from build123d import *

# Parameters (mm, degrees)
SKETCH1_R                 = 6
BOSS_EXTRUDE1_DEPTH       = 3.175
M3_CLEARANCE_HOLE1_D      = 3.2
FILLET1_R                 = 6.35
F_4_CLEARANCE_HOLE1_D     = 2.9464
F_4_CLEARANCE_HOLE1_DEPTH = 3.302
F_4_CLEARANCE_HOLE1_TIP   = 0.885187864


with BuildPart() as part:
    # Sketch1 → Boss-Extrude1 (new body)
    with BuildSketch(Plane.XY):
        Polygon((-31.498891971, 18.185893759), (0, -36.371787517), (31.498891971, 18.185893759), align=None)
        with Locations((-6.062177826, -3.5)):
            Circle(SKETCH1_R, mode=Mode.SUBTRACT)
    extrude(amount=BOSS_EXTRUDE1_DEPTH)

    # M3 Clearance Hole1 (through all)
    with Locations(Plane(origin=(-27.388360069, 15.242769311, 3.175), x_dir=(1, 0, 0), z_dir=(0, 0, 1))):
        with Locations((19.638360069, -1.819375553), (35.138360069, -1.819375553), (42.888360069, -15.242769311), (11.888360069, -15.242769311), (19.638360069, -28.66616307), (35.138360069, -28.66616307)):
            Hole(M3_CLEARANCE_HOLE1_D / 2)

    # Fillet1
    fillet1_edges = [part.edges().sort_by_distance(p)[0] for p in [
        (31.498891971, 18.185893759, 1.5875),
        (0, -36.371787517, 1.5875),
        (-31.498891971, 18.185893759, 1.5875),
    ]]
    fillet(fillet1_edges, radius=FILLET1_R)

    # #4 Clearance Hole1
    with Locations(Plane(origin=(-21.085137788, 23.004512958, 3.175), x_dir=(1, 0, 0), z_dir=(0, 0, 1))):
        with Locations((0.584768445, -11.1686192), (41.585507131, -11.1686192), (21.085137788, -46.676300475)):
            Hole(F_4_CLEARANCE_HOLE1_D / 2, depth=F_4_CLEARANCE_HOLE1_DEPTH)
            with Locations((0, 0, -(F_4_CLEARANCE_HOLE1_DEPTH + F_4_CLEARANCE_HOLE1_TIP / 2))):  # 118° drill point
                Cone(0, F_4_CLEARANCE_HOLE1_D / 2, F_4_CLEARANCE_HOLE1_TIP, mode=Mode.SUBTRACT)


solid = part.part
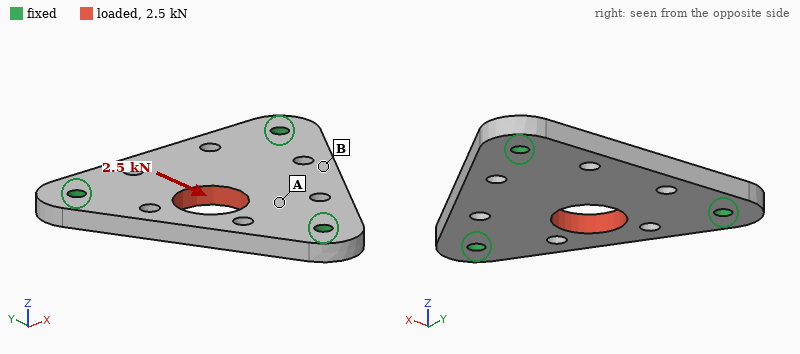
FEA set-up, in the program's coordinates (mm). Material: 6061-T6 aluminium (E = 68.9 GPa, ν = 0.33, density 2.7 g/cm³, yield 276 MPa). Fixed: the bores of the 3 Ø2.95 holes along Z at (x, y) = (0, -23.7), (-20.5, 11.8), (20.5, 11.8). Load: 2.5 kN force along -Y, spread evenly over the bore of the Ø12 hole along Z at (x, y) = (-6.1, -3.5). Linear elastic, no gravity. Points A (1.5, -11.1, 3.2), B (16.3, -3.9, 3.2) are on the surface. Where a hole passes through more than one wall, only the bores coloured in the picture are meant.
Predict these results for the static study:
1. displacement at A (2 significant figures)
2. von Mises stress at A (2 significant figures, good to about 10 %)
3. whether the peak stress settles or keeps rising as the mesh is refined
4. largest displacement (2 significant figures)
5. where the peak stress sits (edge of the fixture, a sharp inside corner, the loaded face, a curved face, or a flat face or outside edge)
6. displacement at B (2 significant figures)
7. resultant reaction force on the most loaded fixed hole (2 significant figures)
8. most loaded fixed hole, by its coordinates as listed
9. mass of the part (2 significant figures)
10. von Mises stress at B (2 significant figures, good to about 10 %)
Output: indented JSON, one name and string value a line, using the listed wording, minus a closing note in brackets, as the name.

{
  "displacement at A": "5.3 µm",
  "von Mises stress at A": "33 MPa",
  "whether the peak stress settles or keeps rising as the mesh is refined": "keeps rising",
  "largest displacement": "13 µm",
  "where the peak stress sits": "edge of the fixture",
  "displacement at B": "3.7 µm",
  "resultant reaction force on the most loaded fixed hole": "1.2 kN",
  "most loaded fixed hole, by its coordinates as listed": "(0, -23.7)",
  "mass of the part": "12 g",
  "von Mises stress at B": "10 MPa"
}
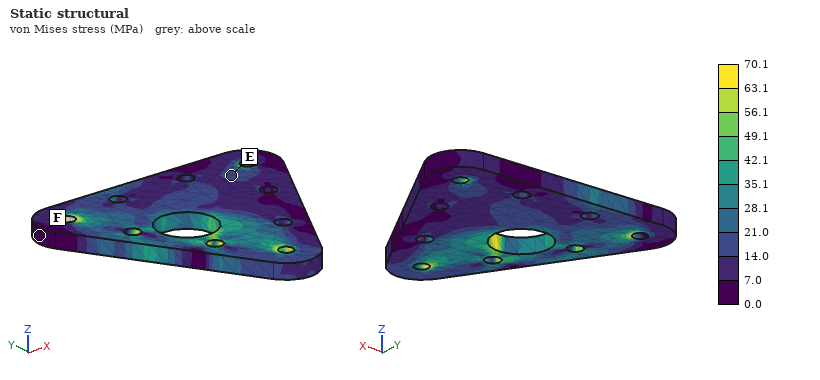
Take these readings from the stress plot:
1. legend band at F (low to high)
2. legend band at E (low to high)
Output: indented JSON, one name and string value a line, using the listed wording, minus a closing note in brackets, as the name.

{
  "legend band at F": "0.0 to 7.0 MPa",
  "legend band at E": "14.0 to 21.0 MPa"
}
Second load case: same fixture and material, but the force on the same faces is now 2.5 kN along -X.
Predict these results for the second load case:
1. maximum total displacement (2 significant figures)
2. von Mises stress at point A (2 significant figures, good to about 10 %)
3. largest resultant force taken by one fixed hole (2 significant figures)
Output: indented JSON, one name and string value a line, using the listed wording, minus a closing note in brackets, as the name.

{
  "maximum total displacement": "19 µm",
  "von Mises stress at point A": "18 MPa",
  "largest resultant force taken by one fixed hole": "980 N"
}
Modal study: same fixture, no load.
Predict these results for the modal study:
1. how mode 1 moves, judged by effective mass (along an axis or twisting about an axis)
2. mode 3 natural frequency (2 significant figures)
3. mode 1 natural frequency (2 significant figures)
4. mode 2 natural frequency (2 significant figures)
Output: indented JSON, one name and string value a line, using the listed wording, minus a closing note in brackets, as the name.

{
  "how mode 1 moves, judged by effective mass": "along Z",
  "mode 3 natural frequency": "12 kHz",
  "mode 1 natural frequency": "8500 Hz",
  "mode 2 natural frequency": "11 kHz"
}
